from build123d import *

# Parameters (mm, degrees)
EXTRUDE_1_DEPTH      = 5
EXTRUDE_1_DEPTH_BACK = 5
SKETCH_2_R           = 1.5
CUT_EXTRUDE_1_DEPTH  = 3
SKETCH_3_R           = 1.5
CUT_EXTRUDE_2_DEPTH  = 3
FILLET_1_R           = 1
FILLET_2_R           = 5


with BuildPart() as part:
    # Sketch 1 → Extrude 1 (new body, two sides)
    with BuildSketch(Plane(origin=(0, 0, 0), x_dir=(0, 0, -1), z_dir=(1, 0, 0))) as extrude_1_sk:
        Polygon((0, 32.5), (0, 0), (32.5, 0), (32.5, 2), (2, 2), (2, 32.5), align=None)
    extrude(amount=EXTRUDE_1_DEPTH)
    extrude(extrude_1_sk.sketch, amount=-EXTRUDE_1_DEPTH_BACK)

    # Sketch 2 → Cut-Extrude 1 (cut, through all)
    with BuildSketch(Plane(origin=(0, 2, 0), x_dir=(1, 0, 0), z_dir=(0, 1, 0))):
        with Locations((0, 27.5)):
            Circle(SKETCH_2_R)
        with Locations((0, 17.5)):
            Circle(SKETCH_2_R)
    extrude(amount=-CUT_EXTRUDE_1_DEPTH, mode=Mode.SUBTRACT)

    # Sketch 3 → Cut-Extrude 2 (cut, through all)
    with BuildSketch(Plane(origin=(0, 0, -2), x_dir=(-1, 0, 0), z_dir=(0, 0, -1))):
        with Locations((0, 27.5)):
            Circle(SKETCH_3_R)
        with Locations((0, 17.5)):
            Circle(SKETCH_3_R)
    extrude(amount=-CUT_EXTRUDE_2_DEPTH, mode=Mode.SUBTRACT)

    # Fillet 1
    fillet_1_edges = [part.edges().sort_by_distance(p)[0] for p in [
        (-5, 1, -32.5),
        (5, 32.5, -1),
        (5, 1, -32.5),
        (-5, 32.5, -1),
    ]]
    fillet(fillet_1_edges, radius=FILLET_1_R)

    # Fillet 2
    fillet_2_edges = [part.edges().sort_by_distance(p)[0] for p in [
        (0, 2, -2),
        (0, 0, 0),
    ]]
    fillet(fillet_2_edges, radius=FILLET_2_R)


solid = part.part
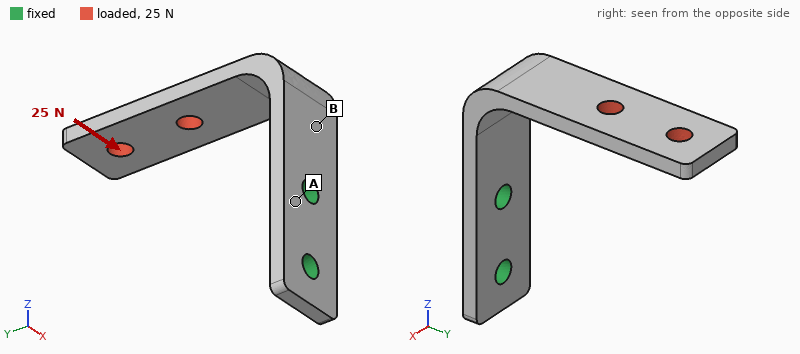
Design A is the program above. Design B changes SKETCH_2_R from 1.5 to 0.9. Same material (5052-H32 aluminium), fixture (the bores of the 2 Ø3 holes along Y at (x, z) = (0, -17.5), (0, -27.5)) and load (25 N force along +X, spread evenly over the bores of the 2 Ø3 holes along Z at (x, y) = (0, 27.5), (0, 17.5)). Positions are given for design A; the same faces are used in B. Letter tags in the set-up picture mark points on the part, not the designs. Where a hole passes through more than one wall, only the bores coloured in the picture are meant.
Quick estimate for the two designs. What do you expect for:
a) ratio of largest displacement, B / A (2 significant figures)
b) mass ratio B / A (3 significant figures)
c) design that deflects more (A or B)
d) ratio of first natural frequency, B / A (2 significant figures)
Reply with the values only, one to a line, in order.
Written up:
1.1
1.02
B
0.97
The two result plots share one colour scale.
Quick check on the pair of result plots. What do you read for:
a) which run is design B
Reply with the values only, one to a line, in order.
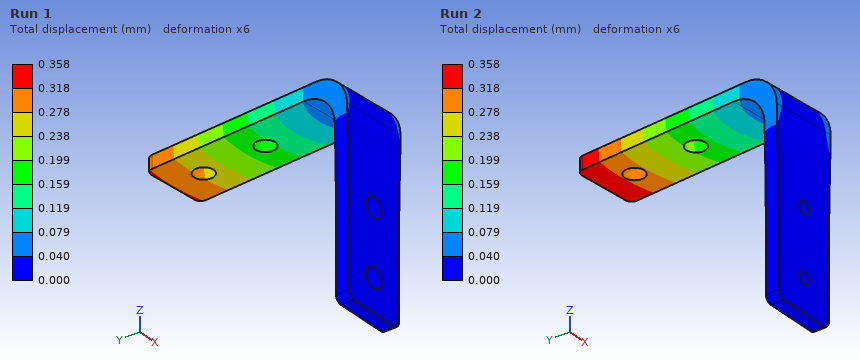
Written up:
Run 2
